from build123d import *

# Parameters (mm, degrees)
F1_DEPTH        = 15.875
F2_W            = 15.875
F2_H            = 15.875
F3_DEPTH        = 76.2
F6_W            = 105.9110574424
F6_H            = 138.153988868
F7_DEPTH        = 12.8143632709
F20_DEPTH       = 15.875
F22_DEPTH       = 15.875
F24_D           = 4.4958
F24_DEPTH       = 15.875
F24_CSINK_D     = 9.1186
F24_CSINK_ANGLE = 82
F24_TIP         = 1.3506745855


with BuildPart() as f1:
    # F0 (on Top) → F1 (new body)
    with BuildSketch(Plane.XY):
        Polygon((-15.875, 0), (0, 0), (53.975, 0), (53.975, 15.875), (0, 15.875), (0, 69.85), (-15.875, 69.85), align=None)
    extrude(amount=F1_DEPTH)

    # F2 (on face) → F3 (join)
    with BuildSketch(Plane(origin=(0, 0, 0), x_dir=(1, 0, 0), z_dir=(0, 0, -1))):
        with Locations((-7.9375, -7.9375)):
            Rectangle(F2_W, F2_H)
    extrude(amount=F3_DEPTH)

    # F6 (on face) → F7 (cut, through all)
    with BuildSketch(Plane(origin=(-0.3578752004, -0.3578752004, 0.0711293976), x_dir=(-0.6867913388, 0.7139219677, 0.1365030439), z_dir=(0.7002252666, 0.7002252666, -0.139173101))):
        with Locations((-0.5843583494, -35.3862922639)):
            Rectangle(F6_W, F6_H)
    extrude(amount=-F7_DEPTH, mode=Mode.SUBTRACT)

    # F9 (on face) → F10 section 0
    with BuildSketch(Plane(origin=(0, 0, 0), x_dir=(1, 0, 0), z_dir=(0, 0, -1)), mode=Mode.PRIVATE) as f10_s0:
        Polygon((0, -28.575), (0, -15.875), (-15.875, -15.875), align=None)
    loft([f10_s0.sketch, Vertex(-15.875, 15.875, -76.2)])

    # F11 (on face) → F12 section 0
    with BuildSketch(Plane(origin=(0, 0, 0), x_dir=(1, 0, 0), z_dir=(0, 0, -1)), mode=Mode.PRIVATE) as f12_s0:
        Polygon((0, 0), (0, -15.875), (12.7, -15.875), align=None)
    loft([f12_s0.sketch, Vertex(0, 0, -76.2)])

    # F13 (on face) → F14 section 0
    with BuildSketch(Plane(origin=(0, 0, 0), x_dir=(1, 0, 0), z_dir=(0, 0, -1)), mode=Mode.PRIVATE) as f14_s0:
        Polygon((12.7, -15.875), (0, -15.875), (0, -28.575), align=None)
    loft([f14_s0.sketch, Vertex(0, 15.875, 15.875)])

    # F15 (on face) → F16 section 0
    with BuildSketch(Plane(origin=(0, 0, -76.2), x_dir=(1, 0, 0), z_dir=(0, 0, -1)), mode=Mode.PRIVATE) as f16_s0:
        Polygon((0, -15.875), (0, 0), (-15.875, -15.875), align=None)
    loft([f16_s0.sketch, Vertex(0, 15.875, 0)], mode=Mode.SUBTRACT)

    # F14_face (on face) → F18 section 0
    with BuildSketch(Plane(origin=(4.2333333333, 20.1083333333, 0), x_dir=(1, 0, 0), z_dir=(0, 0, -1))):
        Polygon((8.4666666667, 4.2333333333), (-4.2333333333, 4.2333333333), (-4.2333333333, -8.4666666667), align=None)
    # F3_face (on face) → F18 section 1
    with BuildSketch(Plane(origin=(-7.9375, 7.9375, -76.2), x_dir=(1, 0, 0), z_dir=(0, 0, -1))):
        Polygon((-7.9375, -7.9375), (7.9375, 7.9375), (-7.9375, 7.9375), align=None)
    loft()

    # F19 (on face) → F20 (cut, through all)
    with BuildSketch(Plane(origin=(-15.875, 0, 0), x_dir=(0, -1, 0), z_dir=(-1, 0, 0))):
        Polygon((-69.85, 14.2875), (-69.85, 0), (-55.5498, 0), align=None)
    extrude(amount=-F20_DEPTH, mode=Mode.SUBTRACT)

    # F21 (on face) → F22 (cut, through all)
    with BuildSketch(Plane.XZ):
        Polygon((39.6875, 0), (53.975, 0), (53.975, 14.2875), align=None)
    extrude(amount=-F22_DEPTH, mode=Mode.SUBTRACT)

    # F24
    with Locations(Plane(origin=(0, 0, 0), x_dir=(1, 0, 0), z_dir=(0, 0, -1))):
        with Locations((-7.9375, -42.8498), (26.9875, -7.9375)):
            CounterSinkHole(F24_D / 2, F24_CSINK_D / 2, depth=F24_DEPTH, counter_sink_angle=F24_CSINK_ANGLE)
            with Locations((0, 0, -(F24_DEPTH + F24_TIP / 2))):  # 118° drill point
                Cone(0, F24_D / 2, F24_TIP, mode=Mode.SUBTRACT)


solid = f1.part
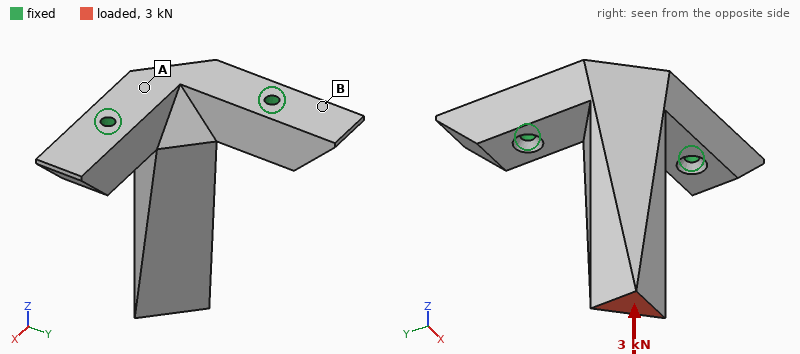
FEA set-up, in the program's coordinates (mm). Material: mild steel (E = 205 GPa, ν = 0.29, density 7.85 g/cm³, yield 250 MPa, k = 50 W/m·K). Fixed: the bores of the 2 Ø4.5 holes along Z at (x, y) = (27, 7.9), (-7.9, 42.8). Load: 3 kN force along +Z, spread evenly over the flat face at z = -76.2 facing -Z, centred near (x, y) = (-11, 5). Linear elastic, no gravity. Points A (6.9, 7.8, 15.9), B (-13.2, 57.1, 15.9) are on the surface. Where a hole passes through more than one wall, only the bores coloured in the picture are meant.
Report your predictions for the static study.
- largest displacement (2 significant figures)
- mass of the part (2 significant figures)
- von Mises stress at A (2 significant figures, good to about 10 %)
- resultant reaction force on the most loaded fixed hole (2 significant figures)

0.14 mm
380 g
30 MPa
1.5 kN
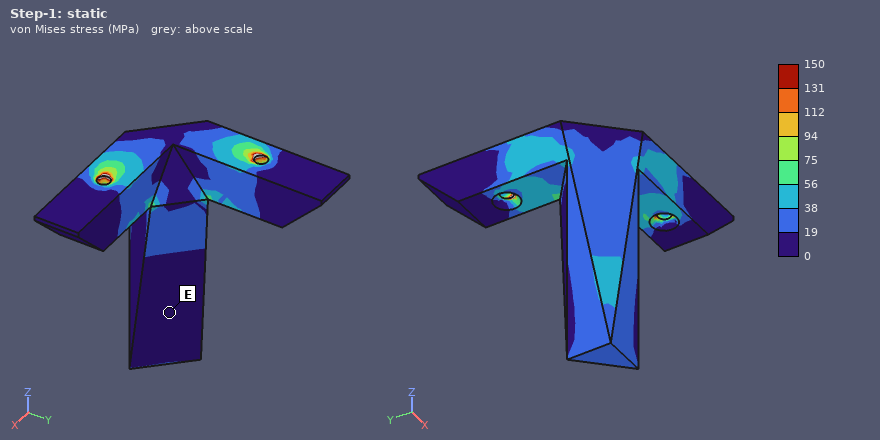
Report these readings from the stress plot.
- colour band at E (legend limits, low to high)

0 to 19 MPa
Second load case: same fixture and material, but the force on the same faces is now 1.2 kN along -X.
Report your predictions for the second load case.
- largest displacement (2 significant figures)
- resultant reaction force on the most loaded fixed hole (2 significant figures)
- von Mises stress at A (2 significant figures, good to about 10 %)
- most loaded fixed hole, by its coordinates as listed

0.20 mm
2.3 kN
47 MPa
(27, 7.9)
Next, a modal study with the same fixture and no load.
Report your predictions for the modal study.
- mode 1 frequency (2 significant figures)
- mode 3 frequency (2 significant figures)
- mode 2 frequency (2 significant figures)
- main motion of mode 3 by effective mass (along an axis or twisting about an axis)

1700 Hz
7200 Hz
2700 Hz
along Z
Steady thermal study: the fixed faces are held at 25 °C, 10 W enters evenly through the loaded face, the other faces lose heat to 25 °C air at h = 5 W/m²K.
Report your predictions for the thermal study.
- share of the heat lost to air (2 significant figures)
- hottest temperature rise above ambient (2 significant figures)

9.0 %
67 K
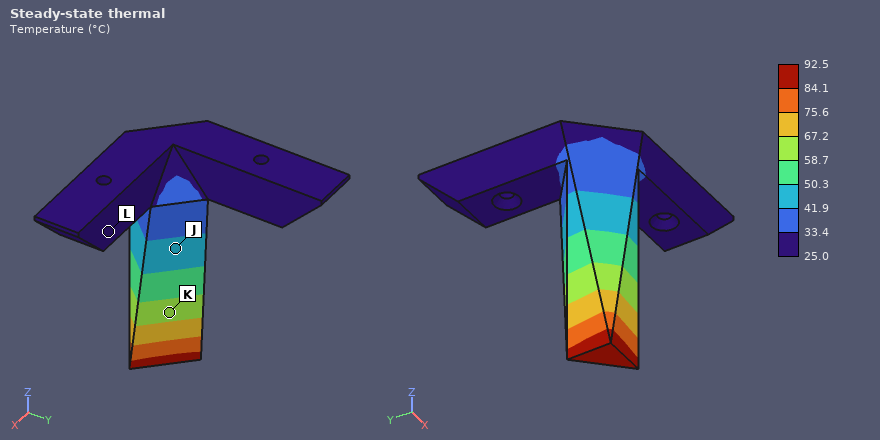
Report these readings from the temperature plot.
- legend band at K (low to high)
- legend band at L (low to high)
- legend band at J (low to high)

58.7 to 67.2 °C
25.0 to 33.4 °C
41.9 to 50.3 °C
